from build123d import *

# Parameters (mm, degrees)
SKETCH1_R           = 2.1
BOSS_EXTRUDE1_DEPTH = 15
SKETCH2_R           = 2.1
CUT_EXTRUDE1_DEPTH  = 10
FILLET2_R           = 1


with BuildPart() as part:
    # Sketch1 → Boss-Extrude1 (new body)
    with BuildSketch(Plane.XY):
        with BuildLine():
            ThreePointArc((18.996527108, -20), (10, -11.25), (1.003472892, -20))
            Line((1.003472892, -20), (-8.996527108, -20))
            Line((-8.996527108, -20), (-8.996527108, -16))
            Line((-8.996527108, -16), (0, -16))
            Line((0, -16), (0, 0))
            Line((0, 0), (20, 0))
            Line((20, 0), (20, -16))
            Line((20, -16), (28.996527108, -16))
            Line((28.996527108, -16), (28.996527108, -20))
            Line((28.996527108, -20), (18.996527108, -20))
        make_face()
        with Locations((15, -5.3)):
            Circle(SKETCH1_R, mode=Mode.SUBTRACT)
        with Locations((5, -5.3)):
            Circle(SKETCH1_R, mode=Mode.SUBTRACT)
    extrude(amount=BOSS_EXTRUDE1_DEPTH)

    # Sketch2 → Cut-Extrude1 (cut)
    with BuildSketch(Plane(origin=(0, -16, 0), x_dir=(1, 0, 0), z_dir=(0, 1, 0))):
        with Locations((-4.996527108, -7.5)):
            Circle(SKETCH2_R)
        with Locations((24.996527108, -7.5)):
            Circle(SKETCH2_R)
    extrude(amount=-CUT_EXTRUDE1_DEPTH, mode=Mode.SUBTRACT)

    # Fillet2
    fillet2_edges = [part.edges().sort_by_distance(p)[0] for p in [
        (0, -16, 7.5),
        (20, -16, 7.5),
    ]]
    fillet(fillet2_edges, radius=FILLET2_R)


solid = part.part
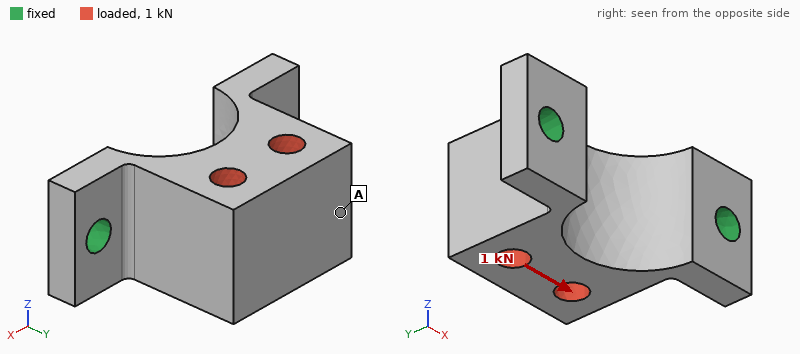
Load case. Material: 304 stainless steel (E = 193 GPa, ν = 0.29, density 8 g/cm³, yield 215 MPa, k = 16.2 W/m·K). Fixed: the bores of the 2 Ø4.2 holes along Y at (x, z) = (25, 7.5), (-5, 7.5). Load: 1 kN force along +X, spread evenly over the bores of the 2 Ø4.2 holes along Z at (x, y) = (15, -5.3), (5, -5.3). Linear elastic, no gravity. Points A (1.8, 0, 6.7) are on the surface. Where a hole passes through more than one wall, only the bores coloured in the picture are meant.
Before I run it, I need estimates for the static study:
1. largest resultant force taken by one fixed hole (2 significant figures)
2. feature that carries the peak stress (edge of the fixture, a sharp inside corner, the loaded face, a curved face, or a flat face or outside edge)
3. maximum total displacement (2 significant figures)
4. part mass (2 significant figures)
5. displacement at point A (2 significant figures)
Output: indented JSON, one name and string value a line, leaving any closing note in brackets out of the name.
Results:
{
  "largest resultant force taken by one fixed hole": "730 N",
  "feature that carries the peak stress": "a curved face",
  "maximum total displacement": "4.3 µm",
  "part mass": "38 g",
  "displacement at point A": "4.2 µm"
}
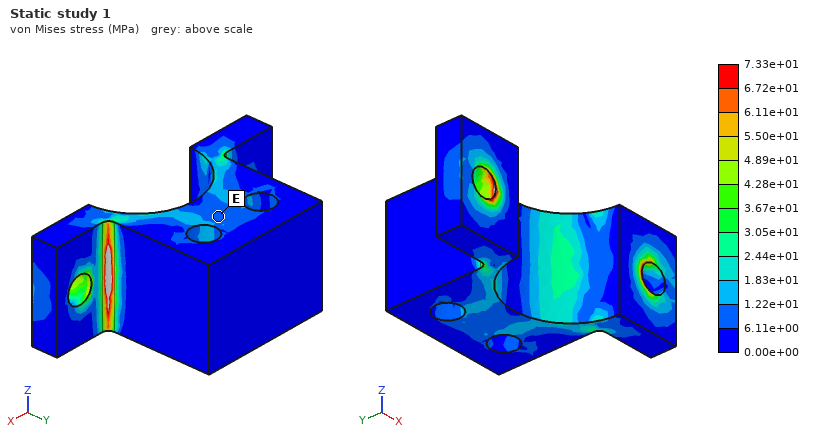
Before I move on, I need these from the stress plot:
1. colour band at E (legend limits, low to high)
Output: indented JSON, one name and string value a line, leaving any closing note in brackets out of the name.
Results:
{
  "colour band at E": "6.11e+00 to 1.22e+01 MPa"
}
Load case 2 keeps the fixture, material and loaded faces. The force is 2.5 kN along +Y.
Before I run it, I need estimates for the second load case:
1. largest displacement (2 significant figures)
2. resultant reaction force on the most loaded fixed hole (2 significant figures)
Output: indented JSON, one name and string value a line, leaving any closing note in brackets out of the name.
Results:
{
  "largest displacement": "5.4 µm",
  "resultant reaction force on the most loaded fixed hole": "1.4 kN"
}
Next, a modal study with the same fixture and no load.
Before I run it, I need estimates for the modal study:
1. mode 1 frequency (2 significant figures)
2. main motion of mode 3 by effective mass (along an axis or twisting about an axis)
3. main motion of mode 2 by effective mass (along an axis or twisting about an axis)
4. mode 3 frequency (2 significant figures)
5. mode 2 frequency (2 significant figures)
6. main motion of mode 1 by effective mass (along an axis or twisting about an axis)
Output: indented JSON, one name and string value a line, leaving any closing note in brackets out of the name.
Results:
{
  "mode 1 frequency": "6400 Hz",
  "main motion of mode 3 by effective mass": "along Y",
  "main motion of mode 2 by effective mass": "along X",
  "mode 3 frequency": "21 kHz",
  "mode 2 frequency": "17 kHz",
  "main motion of mode 1 by effective mass": "along Z"
}
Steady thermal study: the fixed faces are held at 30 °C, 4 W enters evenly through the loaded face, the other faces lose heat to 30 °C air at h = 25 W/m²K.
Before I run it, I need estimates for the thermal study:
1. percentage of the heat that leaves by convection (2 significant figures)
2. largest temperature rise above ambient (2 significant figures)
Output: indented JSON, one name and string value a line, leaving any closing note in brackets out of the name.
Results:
{
  "percentage of the heat that leaves by convection": "25 %",
  "largest temperature rise above ambient": "29 K"
}
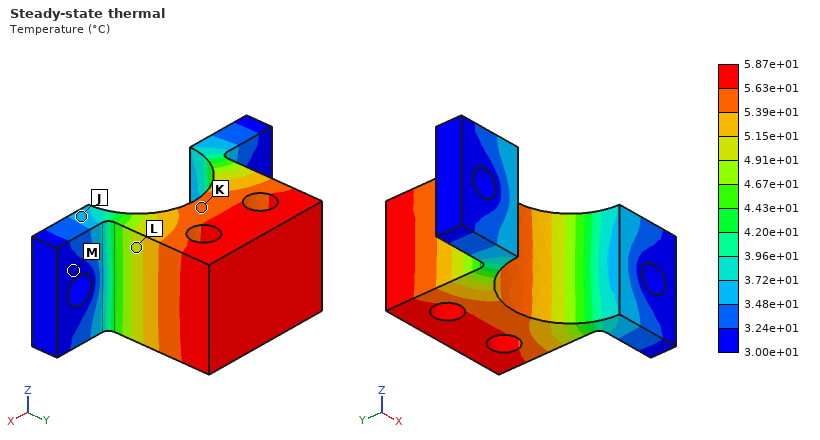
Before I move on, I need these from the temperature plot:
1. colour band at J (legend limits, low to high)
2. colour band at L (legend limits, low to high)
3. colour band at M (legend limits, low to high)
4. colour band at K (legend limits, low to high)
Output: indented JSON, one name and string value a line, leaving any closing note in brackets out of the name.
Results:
{
  "colour band at J": "3.48e+01 to 3.72e+01 °C",
  "colour band at L": "4.91e+01 to 5.15e+01 °C",
  "colour band at M": "3.00e+01 to 3.24e+01 °C",
  "colour band at K": "5.39e+01 to 5.63e+01 °C"
}
